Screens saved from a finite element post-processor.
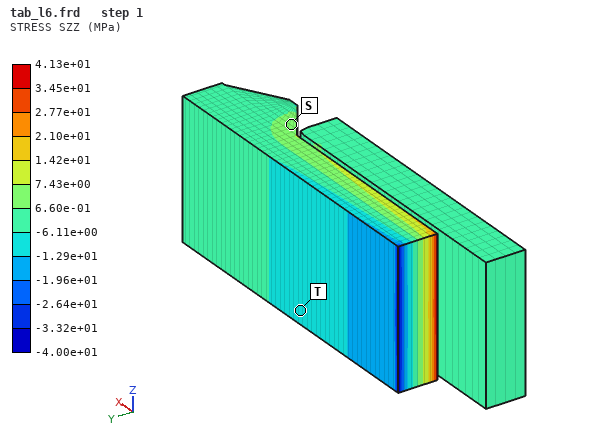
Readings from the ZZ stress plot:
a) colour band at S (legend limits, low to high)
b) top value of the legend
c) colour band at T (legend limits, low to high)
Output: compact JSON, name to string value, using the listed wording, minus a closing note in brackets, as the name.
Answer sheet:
{"colour band at S": "6.60e-01 to 7.43e+00 MPa", "top value of the legend": "4.13e+01 MPa", "colour band at T": "-1.29e+01 to -6.11e+00 MPa"}
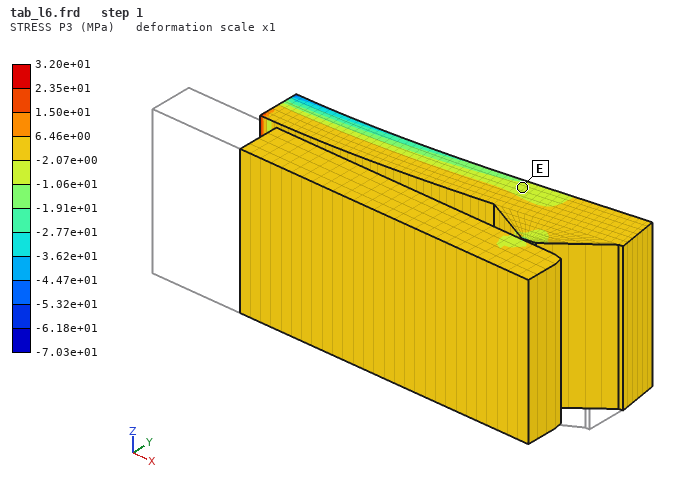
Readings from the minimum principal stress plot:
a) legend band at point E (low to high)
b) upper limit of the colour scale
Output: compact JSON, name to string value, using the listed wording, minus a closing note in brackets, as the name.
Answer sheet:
{"legend band at point E": "-1.06e+01 to -2.07e+00 MPa", "upper limit of the colour scale": "3.20e+01 MPa"}
